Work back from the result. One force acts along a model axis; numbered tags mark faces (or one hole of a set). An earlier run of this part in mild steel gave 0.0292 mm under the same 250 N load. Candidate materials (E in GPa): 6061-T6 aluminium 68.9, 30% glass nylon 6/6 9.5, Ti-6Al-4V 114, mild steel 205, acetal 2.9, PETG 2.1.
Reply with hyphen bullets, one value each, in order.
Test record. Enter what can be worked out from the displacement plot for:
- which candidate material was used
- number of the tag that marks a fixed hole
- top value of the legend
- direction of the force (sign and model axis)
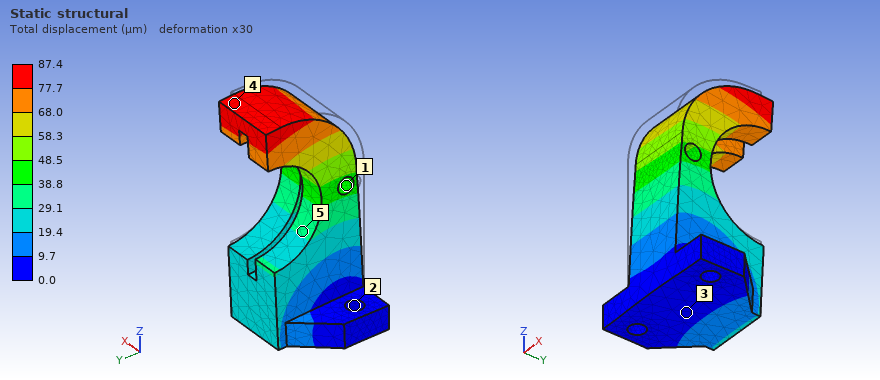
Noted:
- 6061-T6 aluminium
- 2
- 87.4 µm
- +Y
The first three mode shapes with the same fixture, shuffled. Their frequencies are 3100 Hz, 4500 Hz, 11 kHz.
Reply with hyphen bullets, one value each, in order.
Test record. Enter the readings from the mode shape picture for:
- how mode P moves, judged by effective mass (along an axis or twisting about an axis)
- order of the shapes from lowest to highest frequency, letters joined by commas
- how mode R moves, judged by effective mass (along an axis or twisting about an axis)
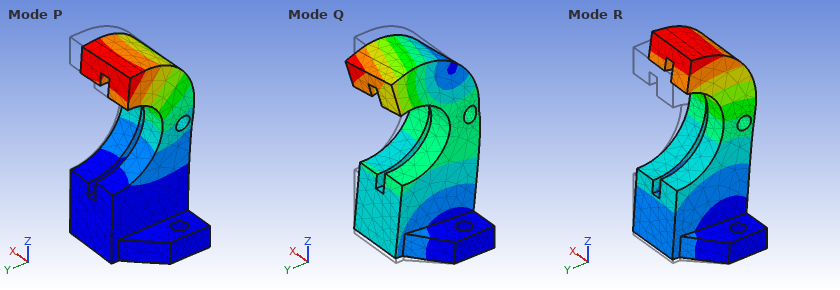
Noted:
- along X
- R, P, Q
- along Y
